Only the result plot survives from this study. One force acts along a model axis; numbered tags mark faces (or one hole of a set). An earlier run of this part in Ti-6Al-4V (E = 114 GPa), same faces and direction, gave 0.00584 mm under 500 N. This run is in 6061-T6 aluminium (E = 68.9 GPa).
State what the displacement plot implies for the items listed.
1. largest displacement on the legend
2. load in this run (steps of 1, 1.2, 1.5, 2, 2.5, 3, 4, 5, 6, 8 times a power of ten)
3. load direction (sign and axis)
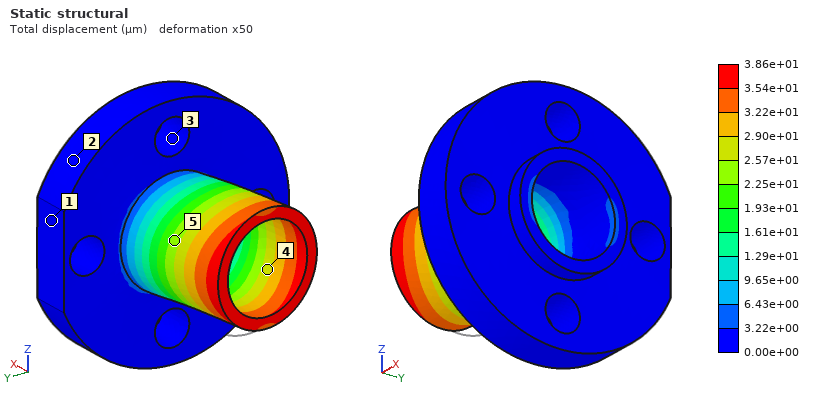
3.86e+01 µm
2 kN
-Y
